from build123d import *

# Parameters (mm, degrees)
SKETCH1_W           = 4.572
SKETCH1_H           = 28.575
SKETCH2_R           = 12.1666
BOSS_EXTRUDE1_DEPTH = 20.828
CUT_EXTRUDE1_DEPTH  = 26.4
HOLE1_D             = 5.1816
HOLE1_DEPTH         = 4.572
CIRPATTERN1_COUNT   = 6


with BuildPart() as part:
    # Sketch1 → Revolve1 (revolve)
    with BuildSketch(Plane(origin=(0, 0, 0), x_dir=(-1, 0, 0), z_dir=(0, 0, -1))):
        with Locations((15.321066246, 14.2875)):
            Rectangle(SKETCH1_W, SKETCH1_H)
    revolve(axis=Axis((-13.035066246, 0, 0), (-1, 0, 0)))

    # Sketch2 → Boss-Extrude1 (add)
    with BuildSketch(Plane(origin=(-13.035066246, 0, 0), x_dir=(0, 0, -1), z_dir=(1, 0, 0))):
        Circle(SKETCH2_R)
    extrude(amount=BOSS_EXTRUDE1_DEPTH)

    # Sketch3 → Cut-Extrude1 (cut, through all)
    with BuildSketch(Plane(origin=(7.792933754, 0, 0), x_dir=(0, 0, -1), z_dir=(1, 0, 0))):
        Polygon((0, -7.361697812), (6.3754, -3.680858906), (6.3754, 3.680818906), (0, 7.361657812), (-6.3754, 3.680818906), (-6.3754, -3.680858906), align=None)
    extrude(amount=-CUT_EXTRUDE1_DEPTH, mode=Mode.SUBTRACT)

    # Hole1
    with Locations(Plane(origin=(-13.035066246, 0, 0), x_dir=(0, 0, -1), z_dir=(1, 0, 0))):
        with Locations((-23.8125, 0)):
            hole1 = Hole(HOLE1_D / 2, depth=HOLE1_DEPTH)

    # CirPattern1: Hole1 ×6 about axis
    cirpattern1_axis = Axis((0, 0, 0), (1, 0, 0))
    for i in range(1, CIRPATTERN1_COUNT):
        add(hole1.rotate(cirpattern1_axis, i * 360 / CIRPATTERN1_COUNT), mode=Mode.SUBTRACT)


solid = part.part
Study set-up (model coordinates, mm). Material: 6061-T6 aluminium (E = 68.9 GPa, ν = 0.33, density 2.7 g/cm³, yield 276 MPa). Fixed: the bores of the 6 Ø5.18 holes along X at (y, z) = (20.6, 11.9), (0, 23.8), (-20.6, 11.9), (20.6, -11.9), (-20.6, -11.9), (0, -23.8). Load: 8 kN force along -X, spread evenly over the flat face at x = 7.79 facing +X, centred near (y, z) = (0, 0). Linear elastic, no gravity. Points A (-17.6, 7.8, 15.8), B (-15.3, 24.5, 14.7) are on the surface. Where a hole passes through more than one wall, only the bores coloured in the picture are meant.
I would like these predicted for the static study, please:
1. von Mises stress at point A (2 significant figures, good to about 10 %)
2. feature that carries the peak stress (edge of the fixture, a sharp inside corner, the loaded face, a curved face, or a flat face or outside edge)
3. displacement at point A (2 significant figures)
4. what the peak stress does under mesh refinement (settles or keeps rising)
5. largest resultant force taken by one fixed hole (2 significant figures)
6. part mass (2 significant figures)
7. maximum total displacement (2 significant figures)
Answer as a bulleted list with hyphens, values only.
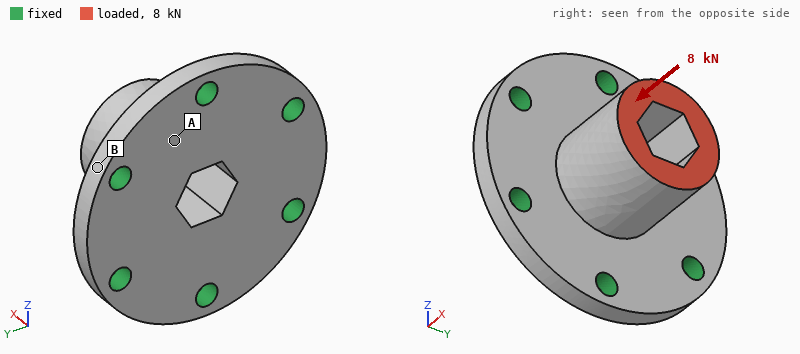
- 46 MPa
- edge of the fixture
- 19 µm
- keeps rising
- 1.5 kN
- 47 g
- 47 µm
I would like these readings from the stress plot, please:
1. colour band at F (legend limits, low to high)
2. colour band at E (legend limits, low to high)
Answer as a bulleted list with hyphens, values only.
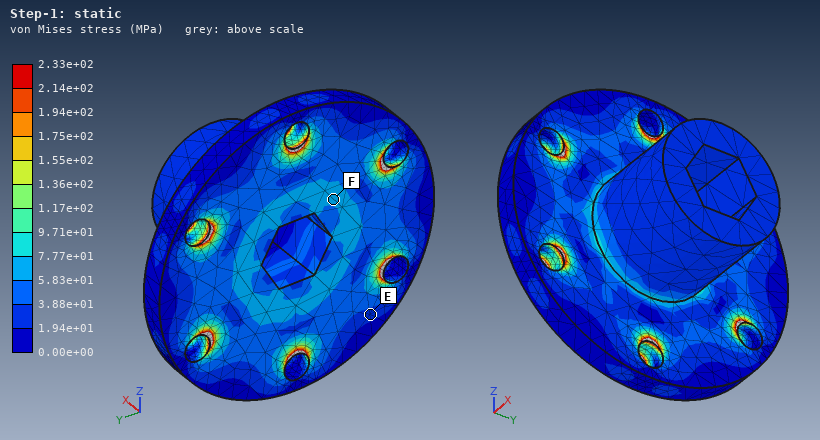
- 5.83e+01 to 7.77e+01 MPa
- 1.94e+01 to 3.88e+01 MPa
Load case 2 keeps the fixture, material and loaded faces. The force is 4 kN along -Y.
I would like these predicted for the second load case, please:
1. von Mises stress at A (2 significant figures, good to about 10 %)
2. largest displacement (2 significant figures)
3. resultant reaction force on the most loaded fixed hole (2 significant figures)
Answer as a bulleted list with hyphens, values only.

- 38 MPa
- 0.11 mm
- 1.7 kN
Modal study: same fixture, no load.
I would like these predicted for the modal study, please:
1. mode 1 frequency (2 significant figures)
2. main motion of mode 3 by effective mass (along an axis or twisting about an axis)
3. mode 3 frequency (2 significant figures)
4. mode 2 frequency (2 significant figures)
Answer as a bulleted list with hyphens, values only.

- 12 kHz
- along X
- 14 kHz
- 12 kHz
